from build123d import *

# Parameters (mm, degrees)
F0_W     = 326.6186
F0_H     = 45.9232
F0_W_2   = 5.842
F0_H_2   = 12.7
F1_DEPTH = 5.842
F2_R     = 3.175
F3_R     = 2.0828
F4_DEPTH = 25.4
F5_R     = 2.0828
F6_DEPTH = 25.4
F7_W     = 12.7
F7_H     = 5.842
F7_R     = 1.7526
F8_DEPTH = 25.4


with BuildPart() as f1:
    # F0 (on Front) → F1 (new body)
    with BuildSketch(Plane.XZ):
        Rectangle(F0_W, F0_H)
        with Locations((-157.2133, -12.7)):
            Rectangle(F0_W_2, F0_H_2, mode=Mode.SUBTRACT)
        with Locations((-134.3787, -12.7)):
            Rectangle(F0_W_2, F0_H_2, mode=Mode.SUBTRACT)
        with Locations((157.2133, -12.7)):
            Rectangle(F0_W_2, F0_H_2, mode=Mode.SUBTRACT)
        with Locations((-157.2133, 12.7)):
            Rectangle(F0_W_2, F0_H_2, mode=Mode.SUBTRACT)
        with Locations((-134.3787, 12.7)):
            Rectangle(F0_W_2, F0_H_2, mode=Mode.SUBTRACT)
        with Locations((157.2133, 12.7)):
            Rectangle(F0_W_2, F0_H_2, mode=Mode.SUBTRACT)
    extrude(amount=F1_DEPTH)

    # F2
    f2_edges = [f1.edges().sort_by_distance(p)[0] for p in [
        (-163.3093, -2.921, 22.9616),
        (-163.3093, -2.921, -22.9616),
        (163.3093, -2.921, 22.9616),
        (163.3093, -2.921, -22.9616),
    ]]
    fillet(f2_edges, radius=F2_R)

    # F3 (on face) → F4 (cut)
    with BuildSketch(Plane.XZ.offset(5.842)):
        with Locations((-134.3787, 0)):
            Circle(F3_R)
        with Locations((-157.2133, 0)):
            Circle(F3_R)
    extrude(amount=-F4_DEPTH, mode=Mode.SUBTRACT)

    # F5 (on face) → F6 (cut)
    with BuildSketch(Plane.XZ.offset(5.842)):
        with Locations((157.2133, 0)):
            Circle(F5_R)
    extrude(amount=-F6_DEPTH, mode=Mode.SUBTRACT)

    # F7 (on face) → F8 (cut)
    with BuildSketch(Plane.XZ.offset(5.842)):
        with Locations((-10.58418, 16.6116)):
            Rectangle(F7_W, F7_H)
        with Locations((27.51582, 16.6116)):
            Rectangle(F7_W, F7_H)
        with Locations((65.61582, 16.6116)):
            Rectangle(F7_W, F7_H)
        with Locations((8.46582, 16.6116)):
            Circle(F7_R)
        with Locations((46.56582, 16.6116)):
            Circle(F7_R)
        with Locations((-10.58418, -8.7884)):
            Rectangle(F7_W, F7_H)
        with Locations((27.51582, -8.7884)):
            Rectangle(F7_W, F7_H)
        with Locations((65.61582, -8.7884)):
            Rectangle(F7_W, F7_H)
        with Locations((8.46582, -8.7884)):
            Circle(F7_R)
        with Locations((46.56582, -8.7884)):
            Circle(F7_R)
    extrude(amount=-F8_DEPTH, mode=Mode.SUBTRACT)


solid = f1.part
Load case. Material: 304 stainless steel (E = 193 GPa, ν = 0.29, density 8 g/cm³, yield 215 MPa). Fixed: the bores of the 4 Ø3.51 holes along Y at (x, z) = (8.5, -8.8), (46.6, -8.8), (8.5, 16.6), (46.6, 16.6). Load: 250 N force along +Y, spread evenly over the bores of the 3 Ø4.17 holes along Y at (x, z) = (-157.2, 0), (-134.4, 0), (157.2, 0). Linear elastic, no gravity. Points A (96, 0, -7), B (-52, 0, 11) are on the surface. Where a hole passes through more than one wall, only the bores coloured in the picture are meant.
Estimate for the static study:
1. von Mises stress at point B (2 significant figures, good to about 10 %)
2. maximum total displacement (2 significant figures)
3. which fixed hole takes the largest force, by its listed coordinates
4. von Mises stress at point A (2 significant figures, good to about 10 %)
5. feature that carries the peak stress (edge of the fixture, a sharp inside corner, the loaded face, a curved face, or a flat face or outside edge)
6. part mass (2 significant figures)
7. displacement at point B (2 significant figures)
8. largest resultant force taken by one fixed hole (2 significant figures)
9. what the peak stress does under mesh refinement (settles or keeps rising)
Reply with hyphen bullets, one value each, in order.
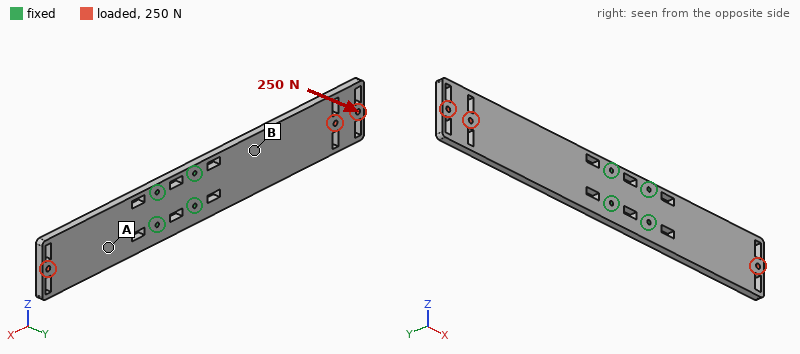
- 60 MPa
- 1.8 mm
- (8.5, -8.8)
- 19 MPa
- edge of the fixture
- 660 g
- 0.33 mm
- 210 N
- keeps rising
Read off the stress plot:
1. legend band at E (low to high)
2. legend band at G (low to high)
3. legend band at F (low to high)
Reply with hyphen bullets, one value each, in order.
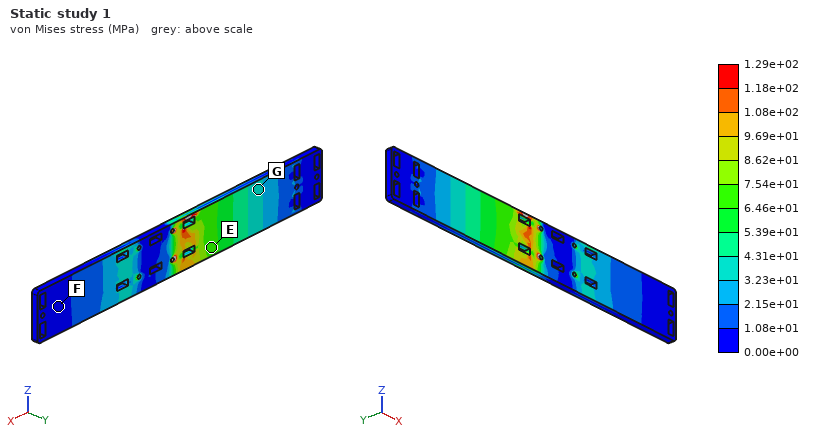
- 6.46e+01 to 7.54e+01 MPa
- 3.23e+01 to 4.31e+01 MPa
- 0.00e+00 to 1.08e+01 MPa
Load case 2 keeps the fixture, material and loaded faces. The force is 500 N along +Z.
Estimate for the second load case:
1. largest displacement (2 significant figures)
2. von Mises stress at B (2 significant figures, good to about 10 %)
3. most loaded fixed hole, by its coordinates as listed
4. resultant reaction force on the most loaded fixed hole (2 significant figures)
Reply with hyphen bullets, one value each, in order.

- 70 µm
- 7.6 MPa
- (8.5, 16.6)
- 1.5 kN
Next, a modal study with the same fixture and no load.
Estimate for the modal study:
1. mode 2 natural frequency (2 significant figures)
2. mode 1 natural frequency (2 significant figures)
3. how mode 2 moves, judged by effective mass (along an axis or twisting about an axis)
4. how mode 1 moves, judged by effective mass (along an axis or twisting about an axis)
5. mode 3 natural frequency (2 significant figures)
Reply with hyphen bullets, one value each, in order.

- 330 Hz
- 160 Hz
- along Y
- along Y
- 980 Hz
